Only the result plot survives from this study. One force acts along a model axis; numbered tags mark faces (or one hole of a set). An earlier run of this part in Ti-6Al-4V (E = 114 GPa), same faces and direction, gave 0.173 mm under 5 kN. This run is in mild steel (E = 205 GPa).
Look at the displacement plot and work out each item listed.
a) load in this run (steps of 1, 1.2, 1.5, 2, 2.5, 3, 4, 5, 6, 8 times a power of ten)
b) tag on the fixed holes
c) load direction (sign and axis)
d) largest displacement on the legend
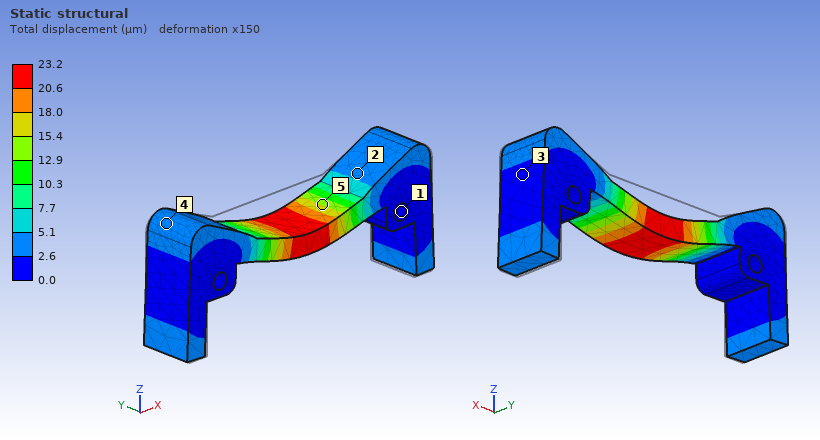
1.2 kN
1
-Z
23.2 µm
